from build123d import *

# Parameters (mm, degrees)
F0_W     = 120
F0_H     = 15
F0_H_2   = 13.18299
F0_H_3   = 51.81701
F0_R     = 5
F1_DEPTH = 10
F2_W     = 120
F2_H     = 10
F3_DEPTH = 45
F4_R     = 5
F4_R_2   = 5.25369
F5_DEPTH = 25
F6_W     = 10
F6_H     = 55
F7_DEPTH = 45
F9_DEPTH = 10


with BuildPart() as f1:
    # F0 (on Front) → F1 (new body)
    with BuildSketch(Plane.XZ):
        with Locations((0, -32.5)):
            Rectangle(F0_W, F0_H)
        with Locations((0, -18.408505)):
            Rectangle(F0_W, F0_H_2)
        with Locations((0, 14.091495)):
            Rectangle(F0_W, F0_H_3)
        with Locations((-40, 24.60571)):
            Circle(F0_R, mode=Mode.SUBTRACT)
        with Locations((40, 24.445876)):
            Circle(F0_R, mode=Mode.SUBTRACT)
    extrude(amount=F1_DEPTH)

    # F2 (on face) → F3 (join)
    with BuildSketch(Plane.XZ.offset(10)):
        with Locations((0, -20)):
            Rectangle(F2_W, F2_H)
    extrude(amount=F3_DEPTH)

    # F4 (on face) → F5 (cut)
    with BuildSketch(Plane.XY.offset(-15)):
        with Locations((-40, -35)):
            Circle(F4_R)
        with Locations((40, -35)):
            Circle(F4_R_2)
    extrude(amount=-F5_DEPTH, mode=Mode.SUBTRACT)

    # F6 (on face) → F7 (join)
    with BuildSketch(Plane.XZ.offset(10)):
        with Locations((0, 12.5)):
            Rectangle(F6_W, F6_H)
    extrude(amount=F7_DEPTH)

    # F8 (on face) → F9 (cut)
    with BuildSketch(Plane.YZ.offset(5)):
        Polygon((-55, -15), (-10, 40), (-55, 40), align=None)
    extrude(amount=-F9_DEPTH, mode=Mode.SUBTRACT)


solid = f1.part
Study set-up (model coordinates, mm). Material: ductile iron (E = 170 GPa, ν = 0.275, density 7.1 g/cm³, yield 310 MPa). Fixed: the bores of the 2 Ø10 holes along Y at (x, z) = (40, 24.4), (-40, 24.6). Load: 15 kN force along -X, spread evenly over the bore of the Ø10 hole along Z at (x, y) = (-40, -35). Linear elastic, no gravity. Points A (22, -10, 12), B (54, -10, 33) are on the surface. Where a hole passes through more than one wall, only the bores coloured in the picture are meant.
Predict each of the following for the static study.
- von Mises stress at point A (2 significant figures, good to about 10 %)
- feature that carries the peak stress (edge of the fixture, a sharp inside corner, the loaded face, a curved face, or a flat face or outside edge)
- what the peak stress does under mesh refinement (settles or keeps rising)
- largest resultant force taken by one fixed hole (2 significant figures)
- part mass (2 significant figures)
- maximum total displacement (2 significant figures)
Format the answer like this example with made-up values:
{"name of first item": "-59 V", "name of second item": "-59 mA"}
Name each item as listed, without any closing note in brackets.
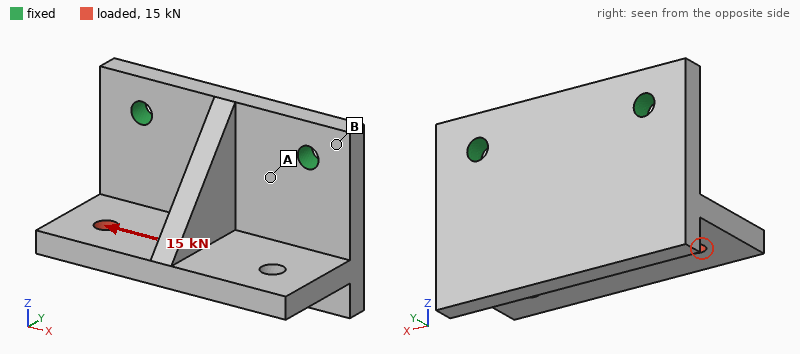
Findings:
{"von Mises stress at point A": "79 MPa", "feature that carries the peak stress": "edge of the fixture", "what the peak stress does under mesh refinement": "keeps rising", "largest resultant force taken by one fixed hole": "12 kN", "part mass": "1.1 kg", "maximum total displacement": "0.16 mm"}
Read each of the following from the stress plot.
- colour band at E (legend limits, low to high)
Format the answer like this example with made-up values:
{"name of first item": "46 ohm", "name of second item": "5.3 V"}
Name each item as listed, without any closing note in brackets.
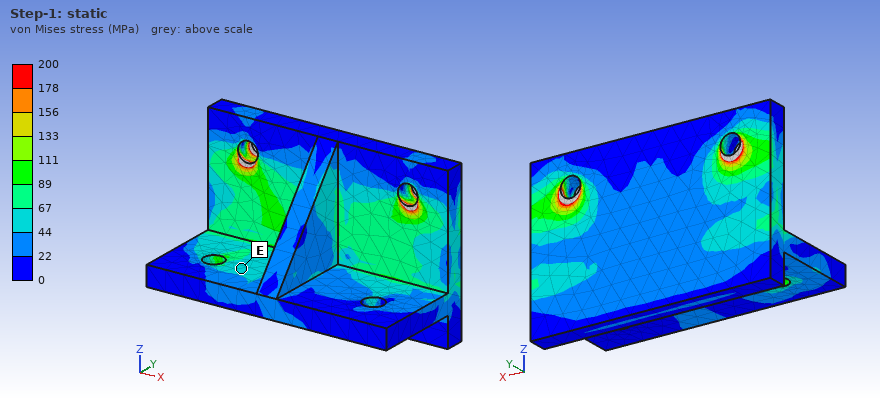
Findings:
{"colour band at E": "44 to 67 MPa"}
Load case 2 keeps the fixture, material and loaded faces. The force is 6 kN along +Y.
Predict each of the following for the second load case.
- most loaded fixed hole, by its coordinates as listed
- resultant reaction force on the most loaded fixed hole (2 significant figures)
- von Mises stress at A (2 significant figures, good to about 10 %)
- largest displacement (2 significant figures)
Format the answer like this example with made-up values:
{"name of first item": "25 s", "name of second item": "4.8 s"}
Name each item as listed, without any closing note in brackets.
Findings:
{"most loaded fixed hole, by its coordinates as listed": "(-40, 24.6)", "resultant reaction force on the most loaded fixed hole": "5.9 kN", "von Mises stress at A": "51 MPa", "largest displacement": "0.26 mm"}
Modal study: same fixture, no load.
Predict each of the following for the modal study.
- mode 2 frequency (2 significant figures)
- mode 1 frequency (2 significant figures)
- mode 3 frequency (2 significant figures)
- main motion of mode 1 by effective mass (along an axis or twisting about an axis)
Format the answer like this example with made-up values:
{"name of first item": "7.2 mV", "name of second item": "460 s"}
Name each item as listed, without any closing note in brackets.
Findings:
{"mode 2 frequency": "2100 Hz", "mode 1 frequency": "1200 Hz", "mode 3 frequency": "4100 Hz", "main motion of mode 1 by effective mass": "along Y"}
